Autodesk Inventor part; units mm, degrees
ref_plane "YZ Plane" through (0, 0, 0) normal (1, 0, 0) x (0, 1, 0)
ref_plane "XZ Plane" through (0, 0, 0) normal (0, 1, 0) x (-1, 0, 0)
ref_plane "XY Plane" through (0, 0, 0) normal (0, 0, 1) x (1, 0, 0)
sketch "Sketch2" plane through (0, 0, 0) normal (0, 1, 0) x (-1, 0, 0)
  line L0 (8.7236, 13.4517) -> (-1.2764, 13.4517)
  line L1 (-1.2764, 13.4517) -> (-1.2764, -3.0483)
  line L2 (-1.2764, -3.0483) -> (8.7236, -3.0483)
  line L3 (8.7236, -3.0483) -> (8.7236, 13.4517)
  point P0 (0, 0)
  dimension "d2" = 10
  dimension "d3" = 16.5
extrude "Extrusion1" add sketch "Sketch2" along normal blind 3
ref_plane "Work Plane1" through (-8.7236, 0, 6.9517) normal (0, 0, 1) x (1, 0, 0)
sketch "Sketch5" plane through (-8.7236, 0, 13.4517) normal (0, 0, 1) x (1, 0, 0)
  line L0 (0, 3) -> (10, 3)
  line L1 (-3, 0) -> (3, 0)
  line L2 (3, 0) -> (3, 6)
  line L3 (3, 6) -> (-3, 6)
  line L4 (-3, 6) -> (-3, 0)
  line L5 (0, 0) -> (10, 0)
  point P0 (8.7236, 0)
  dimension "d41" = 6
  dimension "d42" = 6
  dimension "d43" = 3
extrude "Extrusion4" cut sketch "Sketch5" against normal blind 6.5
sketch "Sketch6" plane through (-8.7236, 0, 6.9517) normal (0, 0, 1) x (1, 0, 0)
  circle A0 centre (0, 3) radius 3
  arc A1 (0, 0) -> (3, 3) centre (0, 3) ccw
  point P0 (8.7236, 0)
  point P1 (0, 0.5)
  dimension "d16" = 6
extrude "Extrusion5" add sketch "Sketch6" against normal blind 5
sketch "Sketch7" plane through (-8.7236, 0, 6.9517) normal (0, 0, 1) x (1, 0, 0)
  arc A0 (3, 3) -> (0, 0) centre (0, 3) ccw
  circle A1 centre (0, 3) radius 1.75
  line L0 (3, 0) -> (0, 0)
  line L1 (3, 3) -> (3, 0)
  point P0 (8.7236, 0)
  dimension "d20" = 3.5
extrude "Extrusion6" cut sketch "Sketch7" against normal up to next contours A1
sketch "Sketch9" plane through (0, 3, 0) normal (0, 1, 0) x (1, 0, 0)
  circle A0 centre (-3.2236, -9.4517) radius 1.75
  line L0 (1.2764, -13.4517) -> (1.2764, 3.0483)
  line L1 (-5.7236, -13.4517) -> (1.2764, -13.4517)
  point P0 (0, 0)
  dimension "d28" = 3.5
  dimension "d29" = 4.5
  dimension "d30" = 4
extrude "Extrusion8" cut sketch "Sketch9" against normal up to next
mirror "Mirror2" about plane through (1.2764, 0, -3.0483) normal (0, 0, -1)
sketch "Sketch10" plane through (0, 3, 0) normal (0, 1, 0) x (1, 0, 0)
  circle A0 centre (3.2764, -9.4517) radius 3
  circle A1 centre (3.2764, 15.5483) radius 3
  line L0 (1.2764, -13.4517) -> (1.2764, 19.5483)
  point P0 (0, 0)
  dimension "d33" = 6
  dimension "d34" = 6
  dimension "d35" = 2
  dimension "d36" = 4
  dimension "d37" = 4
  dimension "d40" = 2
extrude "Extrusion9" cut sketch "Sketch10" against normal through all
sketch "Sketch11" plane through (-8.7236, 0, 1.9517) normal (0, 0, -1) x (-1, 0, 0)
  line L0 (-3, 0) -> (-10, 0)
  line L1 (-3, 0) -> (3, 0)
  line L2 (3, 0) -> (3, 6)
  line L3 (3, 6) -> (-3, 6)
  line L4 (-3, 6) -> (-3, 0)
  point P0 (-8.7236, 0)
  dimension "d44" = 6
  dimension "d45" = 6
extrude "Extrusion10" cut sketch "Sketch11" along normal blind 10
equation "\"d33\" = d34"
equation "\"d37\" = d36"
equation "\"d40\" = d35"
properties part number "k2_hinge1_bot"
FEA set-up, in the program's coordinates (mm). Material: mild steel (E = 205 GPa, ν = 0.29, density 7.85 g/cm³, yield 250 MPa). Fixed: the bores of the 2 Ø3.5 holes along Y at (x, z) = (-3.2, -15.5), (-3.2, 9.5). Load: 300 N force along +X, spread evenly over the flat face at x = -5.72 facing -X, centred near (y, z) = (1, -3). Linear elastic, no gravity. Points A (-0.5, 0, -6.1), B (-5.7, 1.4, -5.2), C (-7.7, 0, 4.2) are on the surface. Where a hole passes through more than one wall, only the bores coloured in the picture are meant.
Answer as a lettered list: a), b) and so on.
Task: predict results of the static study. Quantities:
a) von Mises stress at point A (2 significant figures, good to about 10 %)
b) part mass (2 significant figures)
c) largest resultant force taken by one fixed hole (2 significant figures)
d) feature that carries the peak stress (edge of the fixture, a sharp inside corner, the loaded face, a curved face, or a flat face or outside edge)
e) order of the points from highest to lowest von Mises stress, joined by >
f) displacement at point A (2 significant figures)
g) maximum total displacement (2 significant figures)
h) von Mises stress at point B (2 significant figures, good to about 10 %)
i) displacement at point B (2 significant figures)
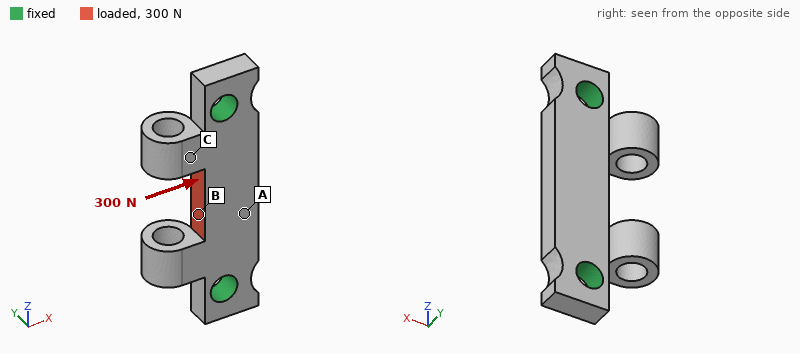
a) 15 MPa
b) 6.5 g
c) 150 N
d) edge of the fixture
e) B > A > C
f) 2.0 µm
g) 2.6 µm
h) 23 MPa
i) 2.2 µm
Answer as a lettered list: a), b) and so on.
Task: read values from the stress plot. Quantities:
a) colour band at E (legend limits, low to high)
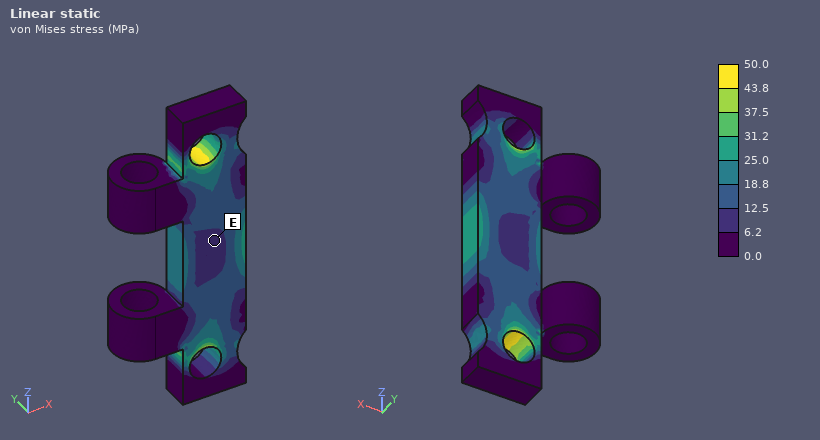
a) 6.2 to 12.5 MPa
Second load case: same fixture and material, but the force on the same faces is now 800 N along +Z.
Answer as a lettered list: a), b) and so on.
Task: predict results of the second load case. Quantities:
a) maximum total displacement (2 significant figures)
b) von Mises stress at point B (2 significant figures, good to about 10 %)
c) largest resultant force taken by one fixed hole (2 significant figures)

a) 1.8 µm
b) 52 MPa
c) 410 N
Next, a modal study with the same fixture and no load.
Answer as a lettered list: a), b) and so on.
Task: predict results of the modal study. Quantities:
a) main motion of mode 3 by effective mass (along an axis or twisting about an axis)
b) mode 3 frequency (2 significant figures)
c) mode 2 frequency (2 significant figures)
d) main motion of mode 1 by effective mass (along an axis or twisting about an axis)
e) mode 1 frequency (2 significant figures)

a) along Y
b) 26 kHz
c) 23 kHz
d) along Y
e) 21 kHz
